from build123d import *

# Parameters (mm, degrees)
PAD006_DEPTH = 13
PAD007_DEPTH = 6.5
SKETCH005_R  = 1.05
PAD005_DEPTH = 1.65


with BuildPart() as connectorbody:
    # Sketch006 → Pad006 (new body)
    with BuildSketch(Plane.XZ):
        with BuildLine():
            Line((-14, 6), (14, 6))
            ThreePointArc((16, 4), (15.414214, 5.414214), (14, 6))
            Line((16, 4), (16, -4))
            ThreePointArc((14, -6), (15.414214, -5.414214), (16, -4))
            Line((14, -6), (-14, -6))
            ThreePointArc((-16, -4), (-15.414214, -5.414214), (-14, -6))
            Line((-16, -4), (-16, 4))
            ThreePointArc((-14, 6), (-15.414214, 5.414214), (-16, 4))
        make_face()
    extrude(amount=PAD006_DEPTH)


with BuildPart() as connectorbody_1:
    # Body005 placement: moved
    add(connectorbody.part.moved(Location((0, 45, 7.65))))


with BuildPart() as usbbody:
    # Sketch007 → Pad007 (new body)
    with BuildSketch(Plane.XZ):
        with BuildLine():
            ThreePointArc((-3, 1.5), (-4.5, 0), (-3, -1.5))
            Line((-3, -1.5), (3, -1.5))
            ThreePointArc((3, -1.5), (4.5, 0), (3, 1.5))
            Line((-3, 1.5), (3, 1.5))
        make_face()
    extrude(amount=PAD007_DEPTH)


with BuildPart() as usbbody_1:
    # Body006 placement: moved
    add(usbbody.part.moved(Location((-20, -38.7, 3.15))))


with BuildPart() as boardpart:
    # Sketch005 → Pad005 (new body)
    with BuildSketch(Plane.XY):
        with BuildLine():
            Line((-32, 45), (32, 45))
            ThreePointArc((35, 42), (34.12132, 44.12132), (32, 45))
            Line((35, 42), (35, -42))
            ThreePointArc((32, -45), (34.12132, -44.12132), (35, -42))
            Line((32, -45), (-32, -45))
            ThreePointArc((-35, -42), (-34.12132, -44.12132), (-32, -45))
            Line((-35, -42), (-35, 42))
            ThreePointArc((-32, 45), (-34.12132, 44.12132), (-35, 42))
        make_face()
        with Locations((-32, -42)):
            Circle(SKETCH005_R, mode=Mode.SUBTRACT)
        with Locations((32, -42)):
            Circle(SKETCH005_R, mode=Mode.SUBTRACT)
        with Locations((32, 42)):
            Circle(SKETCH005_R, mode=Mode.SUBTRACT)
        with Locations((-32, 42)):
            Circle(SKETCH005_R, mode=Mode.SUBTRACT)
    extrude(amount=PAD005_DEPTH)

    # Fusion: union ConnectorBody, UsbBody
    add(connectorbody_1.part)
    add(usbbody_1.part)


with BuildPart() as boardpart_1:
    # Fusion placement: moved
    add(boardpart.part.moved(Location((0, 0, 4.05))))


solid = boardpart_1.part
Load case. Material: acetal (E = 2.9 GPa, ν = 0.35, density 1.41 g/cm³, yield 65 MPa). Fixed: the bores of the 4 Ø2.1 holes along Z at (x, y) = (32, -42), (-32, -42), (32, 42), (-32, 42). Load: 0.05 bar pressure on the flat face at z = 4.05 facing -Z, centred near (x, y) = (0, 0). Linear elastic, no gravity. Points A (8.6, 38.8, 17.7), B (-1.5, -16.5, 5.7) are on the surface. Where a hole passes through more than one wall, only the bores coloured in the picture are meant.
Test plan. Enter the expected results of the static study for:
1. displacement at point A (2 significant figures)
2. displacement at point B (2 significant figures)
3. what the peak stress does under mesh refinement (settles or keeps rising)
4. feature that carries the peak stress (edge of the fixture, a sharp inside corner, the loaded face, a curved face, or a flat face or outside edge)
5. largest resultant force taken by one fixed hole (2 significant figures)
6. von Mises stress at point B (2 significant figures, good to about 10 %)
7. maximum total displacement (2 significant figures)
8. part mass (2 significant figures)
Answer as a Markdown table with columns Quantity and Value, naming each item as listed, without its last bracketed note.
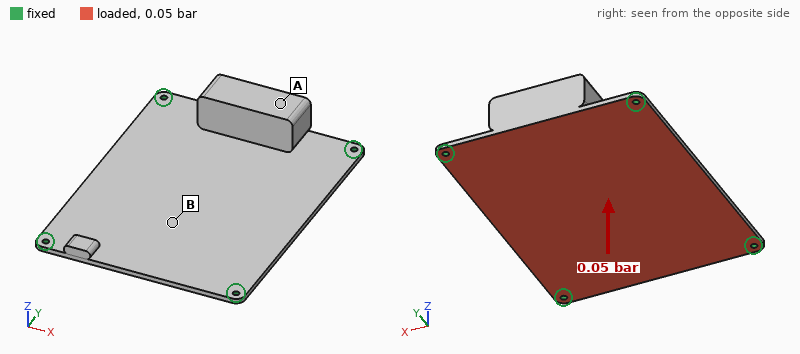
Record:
| Quantity | Value |
|---|---|
| displacement at point A | 0.46 mm |
| displacement at point B | 1.0 mm |
| what the peak stress does under mesh refinement | keeps rising |
| feature that carries the peak stress | edge of the fixture |
| largest resultant force taken by one fixed hole | 8.0 N |
| von Mises stress at point B | 3.2 MPa |
| maximum total displacement | 1.2 mm |
| part mass | 22 g |
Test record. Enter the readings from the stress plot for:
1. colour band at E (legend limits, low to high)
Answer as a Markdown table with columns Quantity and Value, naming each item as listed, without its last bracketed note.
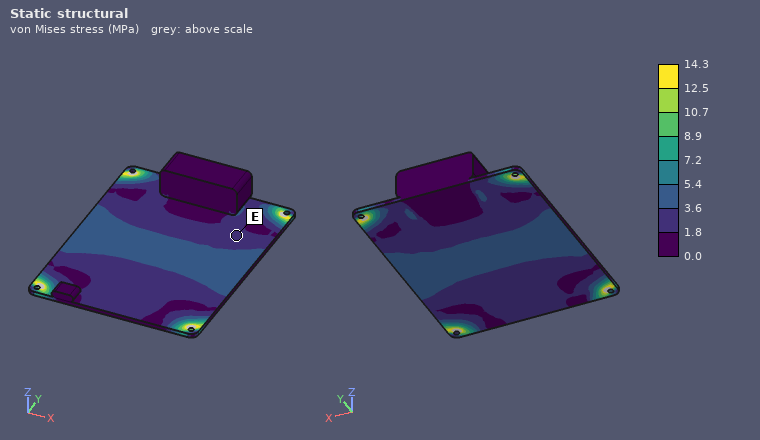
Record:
| Quantity | Value |
|---|---|
| colour band at E | 1.8 to 3.6 MPa |
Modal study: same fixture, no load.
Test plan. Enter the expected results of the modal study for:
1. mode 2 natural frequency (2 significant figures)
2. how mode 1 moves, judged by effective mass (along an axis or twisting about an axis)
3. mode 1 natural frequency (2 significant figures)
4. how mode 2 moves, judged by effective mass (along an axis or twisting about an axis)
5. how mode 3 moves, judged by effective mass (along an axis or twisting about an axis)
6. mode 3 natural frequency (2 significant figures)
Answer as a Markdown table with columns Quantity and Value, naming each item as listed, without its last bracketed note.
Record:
| Quantity | Value |
|---|---|
| mode 2 natural frequency | 410 Hz |
| how mode 1 moves, judged by effective mass | along Z |
| mode 1 natural frequency | 240 Hz |
| how mode 2 moves, judged by effective mass | along Z |
| how mode 3 moves, judged by effective mass | twisting about Y |
| mode 3 natural frequency | 440 Hz |
